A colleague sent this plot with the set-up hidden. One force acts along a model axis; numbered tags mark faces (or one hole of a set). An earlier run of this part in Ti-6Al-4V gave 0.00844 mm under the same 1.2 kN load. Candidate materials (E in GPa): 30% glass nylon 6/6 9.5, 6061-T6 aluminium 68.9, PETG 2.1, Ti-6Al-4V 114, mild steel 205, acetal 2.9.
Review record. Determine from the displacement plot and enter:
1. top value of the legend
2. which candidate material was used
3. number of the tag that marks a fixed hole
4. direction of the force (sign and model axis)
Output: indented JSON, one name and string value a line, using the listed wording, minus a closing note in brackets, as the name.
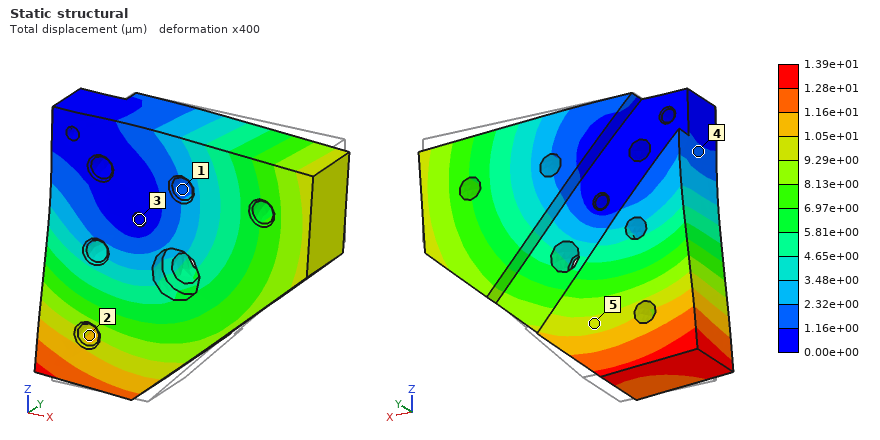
{
  "top value of the legend": "1.39e+01 µm",
  "which candidate material was used": "6061-T6 aluminium",
  "number of the tag that marks a fixed hole": "3",
  "direction of the force": "-X"
}
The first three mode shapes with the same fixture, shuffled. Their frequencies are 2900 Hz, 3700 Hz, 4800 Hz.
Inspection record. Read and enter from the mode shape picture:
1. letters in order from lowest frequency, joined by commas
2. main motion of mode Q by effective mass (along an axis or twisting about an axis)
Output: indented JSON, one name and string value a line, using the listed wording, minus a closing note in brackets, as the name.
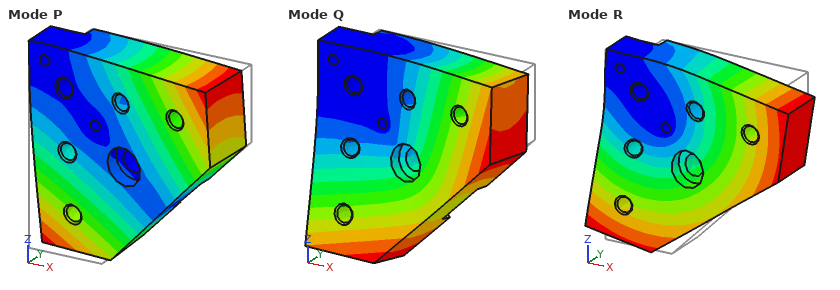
{
  "letters in order from lowest frequency, joined by commas": "P, Q, R",
  "main motion of mode Q by effective mass": "along Y"
}
